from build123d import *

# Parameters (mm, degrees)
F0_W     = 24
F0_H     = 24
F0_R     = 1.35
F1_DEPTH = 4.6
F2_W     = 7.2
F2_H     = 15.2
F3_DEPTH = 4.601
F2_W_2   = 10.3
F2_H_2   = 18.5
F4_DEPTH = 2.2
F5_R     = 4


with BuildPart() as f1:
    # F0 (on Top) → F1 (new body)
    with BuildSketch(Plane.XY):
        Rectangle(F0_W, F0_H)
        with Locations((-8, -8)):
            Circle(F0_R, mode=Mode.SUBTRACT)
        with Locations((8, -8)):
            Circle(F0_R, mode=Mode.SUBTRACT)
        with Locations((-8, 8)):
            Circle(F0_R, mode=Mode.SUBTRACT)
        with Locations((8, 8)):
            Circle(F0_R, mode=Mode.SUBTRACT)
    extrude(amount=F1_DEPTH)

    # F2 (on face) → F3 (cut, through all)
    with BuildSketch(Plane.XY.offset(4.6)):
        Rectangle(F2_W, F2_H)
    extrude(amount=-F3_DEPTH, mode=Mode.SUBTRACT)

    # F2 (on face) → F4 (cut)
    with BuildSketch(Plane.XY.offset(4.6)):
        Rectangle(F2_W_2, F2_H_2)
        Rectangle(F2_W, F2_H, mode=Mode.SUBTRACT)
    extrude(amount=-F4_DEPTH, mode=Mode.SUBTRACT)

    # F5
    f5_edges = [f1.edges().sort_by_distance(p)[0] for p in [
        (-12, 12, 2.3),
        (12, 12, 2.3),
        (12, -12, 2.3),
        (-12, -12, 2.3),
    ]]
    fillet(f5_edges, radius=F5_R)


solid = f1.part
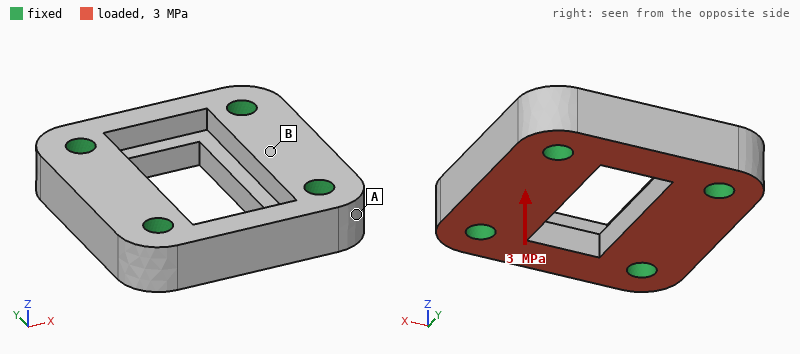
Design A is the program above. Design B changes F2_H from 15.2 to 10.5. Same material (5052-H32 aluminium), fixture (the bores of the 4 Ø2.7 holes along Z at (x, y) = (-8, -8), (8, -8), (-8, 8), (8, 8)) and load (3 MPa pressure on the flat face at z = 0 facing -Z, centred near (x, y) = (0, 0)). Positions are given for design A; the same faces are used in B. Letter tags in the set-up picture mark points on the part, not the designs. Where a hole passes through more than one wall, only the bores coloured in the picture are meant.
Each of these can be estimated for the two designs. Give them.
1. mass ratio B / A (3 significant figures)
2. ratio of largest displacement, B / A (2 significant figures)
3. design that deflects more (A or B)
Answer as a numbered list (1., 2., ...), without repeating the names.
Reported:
1. 1.05
2. 1.3
3. B
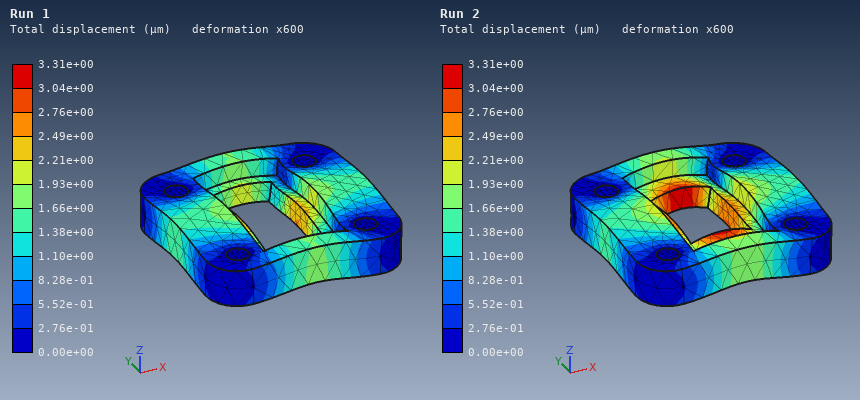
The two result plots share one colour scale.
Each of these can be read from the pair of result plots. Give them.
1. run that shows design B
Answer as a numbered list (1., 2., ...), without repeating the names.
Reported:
1. Run 2
